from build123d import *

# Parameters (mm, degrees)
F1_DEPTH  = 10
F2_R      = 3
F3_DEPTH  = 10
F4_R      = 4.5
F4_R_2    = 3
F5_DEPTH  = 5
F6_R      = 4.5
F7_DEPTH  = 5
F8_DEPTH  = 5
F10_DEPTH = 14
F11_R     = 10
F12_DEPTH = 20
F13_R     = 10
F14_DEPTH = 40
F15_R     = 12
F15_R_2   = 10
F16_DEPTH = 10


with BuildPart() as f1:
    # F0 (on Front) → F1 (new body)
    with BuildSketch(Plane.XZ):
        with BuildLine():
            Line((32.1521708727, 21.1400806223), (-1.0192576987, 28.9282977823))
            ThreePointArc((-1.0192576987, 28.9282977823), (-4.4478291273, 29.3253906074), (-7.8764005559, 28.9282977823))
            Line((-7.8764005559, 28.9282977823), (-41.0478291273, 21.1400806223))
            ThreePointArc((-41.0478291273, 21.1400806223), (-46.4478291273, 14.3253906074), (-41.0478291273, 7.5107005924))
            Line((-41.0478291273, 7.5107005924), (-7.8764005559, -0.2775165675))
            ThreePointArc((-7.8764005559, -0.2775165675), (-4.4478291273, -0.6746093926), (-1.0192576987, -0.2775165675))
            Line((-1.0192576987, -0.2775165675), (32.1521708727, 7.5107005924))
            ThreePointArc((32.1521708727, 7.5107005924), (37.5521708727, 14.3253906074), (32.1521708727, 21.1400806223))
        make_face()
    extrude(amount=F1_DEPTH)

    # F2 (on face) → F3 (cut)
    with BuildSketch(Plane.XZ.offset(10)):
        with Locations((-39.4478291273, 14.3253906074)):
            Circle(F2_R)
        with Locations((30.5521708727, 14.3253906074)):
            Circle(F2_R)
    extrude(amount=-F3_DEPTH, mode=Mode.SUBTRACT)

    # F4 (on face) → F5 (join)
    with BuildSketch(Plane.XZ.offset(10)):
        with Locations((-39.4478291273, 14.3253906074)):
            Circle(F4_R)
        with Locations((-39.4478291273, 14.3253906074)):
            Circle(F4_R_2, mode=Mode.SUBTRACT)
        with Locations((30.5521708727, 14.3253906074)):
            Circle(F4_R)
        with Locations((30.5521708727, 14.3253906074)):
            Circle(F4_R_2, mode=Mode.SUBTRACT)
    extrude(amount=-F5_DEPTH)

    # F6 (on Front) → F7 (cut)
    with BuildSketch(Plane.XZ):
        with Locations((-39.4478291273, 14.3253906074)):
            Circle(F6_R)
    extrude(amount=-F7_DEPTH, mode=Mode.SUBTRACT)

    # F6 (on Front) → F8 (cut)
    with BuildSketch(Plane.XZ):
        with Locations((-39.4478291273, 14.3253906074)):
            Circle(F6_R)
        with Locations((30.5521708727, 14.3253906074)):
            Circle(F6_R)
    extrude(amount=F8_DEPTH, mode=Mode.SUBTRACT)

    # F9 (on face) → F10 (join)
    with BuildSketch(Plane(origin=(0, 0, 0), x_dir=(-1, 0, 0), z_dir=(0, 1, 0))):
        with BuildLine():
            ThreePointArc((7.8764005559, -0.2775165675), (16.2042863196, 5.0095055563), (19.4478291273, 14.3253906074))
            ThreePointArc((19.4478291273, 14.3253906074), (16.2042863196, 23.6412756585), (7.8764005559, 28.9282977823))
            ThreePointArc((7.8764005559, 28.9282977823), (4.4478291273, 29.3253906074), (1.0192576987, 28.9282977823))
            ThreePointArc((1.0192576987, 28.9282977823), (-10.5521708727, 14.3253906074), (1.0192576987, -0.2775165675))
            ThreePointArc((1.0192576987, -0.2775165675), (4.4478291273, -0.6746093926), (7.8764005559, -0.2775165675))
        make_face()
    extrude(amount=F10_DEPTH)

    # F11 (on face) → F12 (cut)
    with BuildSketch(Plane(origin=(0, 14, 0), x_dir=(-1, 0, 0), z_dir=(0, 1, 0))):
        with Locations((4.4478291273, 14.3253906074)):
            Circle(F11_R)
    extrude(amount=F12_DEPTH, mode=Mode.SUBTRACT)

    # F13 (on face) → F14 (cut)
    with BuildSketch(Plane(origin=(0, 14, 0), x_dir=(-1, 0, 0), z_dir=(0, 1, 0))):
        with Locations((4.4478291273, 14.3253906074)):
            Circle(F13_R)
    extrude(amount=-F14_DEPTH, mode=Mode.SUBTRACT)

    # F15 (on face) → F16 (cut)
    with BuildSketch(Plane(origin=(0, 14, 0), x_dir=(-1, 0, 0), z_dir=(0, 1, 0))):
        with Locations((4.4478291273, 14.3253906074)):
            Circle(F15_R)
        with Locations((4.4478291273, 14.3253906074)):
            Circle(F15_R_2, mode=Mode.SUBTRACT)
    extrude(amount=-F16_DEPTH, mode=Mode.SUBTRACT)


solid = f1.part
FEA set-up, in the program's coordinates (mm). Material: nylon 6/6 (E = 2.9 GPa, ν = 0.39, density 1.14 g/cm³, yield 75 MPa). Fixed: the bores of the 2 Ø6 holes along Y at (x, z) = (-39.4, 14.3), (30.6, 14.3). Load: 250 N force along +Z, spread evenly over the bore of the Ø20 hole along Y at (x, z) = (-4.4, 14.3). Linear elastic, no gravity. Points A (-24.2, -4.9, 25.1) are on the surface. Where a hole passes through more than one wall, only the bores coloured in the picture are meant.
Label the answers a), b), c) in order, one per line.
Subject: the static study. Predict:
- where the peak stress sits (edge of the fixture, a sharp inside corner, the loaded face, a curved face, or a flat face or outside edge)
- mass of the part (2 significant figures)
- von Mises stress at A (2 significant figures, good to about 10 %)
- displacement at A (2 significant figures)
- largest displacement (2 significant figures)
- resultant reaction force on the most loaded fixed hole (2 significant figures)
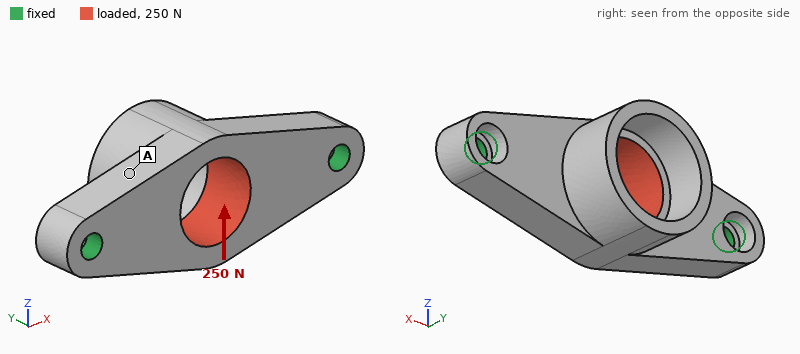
a) edge of the fixture
b) 20 g
c) 1.8 MPa
d) 0.046 mm
e) 0.12 mm
f) 130 N
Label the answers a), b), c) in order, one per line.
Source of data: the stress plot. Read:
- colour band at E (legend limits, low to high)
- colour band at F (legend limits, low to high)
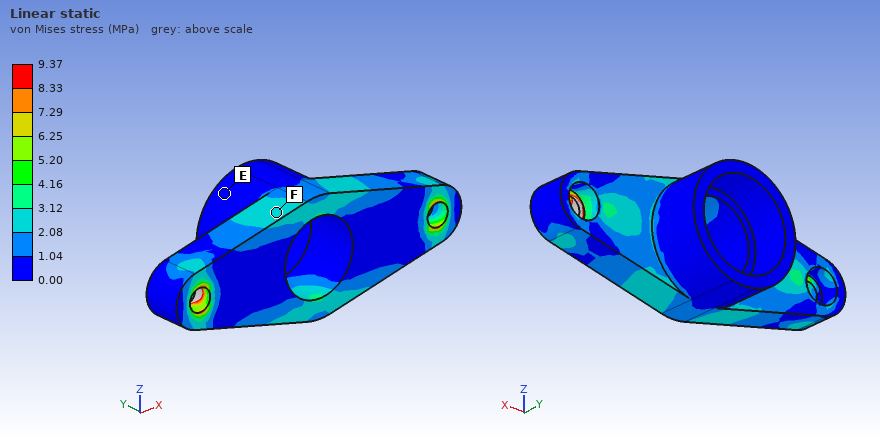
a) 0.00 to 1.04 MPa
b) 2.08 to 3.12 MPa
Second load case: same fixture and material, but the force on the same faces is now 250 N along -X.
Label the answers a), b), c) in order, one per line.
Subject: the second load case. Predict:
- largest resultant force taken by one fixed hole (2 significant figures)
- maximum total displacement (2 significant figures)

a) 130 N
b) 9.7 µm
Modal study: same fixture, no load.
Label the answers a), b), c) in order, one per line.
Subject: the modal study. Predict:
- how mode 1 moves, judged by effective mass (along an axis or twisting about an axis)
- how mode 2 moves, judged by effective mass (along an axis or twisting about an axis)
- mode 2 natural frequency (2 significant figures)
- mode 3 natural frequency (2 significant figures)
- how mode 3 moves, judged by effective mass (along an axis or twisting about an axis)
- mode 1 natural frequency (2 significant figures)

a) along Z
b) along Y
c) 2100 Hz
d) 3900 Hz
e) along Z
f) 1800 Hz
